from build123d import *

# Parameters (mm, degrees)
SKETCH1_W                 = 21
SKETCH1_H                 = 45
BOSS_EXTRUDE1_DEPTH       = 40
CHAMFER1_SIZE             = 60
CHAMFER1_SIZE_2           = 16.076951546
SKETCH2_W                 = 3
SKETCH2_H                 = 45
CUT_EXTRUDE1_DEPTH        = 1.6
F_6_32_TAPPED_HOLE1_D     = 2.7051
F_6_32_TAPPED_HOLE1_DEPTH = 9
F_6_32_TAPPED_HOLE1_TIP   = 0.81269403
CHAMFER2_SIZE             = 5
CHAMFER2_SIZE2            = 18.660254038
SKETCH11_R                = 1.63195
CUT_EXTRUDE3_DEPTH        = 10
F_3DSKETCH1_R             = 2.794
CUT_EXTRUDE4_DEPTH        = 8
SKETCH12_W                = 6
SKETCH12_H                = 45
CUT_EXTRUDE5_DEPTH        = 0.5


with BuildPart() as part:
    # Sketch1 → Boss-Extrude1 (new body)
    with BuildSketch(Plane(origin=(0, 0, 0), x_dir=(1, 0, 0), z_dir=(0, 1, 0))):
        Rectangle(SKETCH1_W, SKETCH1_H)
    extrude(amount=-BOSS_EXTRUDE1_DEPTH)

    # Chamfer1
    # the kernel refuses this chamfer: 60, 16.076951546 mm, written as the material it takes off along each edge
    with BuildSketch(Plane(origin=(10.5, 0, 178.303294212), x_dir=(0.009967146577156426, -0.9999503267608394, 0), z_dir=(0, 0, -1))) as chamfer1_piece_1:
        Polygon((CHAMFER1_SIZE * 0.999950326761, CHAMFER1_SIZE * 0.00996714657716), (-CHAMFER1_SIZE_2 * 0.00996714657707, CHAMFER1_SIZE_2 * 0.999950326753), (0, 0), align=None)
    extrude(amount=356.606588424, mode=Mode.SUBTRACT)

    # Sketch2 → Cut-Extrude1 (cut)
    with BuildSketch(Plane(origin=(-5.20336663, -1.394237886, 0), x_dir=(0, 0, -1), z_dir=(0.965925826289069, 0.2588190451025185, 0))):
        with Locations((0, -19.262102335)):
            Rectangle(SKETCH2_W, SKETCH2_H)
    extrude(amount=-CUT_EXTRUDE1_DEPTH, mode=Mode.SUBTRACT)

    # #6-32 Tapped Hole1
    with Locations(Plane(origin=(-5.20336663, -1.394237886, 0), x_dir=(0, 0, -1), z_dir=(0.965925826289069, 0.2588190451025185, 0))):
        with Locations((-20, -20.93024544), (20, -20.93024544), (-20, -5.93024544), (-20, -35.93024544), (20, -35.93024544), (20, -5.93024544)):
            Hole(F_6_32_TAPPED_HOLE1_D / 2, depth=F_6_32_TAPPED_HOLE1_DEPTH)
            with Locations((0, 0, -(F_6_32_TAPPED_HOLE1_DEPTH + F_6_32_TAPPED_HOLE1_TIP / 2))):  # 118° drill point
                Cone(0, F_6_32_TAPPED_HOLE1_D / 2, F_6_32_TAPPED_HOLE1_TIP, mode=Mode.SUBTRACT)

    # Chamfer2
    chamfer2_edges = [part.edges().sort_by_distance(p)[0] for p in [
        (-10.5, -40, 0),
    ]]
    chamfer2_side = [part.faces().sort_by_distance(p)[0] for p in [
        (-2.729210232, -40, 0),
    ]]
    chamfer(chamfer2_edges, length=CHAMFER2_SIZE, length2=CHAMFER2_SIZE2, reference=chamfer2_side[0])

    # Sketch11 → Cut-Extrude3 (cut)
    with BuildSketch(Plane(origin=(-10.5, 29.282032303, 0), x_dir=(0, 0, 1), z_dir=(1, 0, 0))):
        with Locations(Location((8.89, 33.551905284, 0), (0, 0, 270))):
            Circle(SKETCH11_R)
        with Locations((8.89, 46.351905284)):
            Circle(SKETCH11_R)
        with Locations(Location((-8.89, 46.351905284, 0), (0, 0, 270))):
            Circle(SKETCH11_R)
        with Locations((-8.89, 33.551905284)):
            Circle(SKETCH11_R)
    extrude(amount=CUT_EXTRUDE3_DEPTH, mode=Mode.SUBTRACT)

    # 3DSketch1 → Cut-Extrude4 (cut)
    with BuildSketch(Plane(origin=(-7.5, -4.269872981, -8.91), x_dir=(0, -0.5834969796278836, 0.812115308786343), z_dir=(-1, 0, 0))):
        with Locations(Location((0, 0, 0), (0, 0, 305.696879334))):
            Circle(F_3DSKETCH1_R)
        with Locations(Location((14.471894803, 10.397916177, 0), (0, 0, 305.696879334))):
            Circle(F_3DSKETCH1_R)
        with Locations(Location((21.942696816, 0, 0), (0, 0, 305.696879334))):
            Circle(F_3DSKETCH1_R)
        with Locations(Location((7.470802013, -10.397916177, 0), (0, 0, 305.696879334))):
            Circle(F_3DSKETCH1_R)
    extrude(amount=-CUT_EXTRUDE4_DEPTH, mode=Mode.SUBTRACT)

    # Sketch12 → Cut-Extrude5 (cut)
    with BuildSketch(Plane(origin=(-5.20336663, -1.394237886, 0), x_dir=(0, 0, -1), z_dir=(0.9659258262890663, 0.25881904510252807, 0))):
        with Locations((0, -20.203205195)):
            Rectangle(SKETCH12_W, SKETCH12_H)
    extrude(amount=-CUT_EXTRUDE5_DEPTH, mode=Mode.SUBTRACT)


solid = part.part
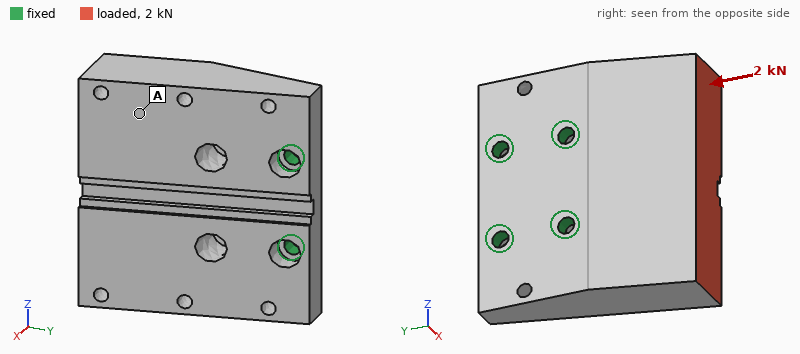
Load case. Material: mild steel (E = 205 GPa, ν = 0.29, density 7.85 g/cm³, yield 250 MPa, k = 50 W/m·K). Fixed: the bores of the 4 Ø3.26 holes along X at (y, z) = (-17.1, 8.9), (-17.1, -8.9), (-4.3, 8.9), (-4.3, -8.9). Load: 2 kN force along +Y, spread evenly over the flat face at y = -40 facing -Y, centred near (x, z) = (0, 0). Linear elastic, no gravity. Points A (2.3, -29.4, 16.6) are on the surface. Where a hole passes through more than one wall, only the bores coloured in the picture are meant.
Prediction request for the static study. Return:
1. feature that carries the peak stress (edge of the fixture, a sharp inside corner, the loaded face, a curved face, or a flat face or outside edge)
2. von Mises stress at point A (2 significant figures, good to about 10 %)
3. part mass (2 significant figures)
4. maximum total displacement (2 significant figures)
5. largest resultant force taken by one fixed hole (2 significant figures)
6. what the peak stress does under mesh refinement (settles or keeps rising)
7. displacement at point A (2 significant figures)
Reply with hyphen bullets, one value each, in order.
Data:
- edge of the fixture
- 11 MPa
- 120 g
- 11 µm
- 860 N
- keeps rising
- 6.5 µm
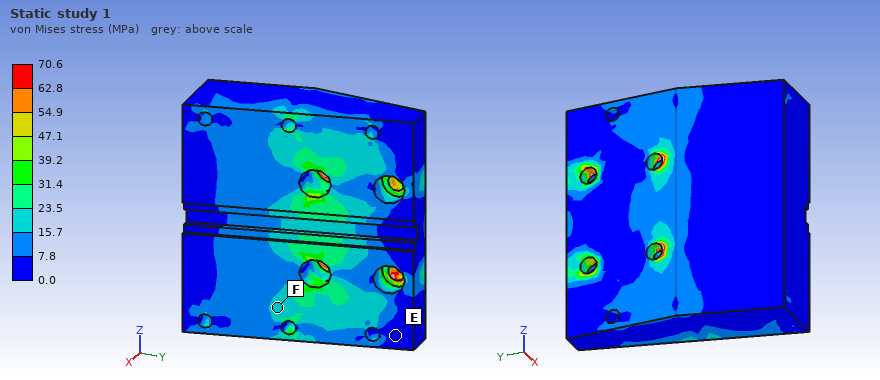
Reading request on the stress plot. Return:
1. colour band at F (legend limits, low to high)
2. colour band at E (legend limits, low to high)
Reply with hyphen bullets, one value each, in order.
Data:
- 15.7 to 23.5 MPa
- 0.0 to 7.8 MPa
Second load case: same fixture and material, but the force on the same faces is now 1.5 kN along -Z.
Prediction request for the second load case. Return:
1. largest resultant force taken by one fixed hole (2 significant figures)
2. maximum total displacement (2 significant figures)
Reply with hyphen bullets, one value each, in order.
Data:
- 1.4 kN
- 6.0 µm
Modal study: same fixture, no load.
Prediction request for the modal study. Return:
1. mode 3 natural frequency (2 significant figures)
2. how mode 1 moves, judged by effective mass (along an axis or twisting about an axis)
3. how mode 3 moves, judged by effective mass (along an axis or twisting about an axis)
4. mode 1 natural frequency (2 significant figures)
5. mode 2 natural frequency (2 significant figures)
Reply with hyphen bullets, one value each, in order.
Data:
- 15 kHz
- along X
- along Z
- 7200 Hz
- 10 kHz
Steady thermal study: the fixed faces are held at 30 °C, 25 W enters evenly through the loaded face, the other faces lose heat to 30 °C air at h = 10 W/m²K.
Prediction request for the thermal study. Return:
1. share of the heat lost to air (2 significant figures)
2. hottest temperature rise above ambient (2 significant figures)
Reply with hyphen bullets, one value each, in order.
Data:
- 3.5 %
- 40 K
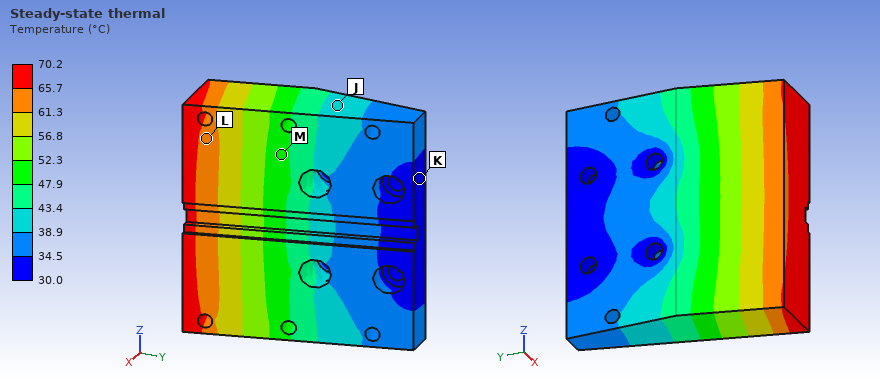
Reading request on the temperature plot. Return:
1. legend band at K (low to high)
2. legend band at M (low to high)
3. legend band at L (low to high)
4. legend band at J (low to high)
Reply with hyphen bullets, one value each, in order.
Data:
- 30.0 to 34.5 °C
- 47.9 to 52.3 °C
- 61.3 to 65.7 °C
- 38.9 to 43.4 °C
